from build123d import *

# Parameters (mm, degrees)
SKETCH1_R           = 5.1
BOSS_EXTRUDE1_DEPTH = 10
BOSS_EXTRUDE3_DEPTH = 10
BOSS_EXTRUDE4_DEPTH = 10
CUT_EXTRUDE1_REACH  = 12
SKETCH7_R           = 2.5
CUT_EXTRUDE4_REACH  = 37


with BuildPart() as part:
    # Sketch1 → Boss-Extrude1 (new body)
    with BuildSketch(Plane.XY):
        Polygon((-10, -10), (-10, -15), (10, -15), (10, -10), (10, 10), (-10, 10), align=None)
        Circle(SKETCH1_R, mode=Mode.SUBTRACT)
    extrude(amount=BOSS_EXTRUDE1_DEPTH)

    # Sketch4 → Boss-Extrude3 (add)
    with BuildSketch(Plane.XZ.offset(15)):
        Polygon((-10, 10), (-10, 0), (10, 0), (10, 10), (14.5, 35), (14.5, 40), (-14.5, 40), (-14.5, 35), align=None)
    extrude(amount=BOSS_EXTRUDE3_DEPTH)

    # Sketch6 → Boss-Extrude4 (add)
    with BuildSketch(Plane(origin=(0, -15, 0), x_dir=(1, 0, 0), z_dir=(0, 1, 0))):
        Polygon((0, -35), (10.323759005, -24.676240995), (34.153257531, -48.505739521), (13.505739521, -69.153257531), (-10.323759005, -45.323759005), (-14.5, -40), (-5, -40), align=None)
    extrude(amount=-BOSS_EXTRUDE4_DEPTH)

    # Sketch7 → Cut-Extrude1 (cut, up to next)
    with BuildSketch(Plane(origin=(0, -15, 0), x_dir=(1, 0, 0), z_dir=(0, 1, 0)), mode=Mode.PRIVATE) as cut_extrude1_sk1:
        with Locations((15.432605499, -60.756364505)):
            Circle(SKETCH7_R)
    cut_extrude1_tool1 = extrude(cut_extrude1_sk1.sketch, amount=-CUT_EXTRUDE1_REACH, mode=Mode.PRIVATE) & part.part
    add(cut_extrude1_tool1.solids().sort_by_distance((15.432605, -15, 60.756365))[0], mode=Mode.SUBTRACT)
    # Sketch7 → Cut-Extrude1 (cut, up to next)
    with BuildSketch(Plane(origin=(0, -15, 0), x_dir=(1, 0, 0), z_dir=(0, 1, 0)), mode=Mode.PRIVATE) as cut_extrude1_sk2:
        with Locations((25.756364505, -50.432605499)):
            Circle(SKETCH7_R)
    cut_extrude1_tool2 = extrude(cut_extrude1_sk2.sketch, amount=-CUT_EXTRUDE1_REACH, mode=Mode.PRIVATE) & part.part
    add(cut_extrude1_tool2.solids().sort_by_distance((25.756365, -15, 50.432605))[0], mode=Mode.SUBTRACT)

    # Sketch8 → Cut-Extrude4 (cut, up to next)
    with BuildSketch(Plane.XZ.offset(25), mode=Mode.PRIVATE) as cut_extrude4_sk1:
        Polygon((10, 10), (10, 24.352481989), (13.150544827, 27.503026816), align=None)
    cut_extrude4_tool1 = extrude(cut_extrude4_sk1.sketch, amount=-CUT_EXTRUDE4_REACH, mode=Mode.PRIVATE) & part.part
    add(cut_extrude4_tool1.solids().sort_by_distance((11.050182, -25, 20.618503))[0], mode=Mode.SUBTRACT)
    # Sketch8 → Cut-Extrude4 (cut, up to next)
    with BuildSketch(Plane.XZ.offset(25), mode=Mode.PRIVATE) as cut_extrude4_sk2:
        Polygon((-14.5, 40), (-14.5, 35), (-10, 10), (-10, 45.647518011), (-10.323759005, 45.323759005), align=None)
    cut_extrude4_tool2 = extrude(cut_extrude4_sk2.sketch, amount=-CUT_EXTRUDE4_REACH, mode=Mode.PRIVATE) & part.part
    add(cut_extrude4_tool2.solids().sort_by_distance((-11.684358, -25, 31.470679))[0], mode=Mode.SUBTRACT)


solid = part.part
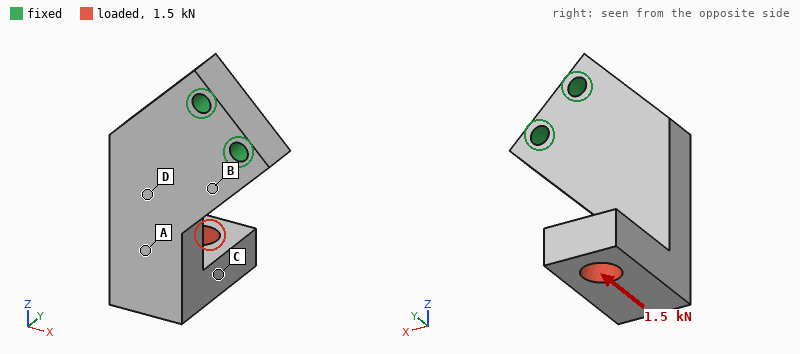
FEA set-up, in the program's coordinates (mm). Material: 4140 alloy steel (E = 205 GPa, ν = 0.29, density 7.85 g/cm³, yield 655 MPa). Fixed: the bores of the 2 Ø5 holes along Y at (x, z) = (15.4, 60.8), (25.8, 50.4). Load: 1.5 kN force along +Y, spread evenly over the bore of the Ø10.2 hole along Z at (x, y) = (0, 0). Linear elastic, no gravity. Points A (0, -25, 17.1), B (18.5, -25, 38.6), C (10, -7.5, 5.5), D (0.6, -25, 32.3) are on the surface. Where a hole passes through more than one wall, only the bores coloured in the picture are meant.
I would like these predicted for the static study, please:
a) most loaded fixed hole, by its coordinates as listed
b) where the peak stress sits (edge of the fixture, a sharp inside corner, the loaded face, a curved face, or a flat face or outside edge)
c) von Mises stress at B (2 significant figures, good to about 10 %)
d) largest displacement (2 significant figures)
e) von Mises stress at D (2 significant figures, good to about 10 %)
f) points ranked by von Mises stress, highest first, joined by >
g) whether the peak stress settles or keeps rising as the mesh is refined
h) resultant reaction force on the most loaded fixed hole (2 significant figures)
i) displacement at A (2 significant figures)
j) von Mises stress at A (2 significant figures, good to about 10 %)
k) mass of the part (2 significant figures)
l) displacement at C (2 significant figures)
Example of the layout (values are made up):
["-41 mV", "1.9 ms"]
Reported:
["(25.8, 50.4)", "edge of the fixture", "140 MPa", "0.26 mm", "98 MPa", "B > D > A > C", "keeps rising", "2.1 kN", "0.12 mm", "54 MPa", "160 g", "0.17 mm"]
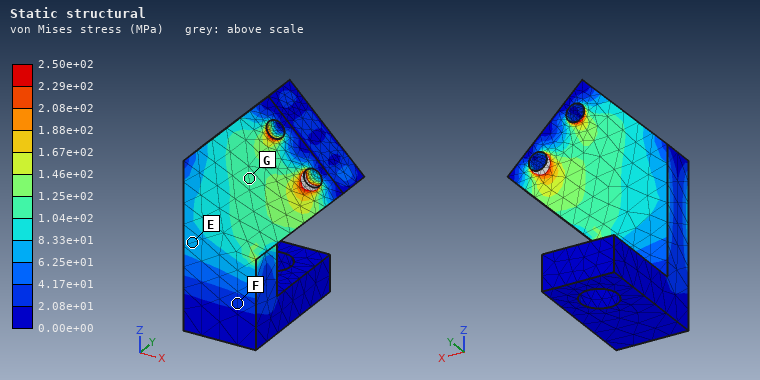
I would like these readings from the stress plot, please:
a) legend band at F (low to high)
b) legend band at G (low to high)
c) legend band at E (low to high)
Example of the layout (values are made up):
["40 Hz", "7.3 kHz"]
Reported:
["2.08e+01 to 4.17e+01 MPa", "1.04e+02 to 1.25e+02 MPa", "6.25e+01 to 8.33e+01 MPa"]
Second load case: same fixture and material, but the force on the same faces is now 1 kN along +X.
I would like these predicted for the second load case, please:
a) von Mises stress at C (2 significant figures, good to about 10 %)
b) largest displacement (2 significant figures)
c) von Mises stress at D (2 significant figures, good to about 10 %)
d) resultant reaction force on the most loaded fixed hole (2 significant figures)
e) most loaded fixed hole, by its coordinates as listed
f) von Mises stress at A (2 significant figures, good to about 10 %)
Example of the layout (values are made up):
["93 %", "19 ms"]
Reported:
["20 MPa", "0.10 mm", "51 MPa", "3.2 kN", "(25.8, 50.4)", "50 MPa"]
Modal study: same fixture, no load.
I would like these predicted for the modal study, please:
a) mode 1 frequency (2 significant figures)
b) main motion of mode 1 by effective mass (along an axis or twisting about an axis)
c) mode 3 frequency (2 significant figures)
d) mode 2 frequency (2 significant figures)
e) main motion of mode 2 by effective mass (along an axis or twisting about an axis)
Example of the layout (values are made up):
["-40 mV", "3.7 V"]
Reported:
["1700 Hz", "along Y", "5700 Hz", "3200 Hz", "along X"]
